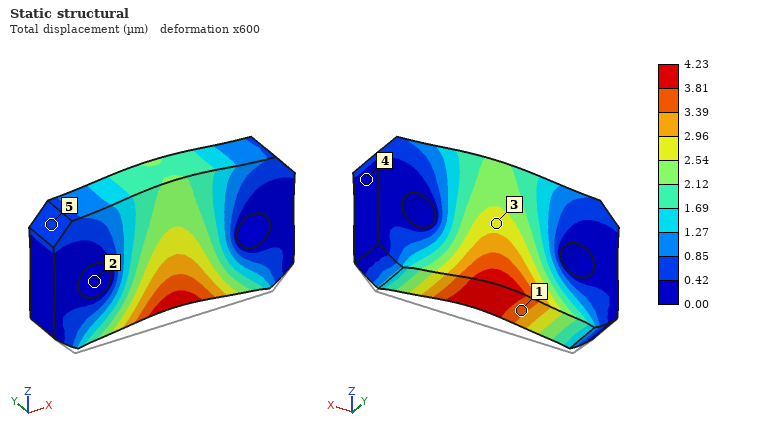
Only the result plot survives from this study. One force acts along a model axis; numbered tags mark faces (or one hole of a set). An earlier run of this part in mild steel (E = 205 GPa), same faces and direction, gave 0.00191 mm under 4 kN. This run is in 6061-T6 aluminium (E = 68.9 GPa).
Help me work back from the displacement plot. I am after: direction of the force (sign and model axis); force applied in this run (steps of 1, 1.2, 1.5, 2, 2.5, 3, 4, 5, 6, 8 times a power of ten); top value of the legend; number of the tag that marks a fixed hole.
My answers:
+Z
3 kN
4.23 µm
2
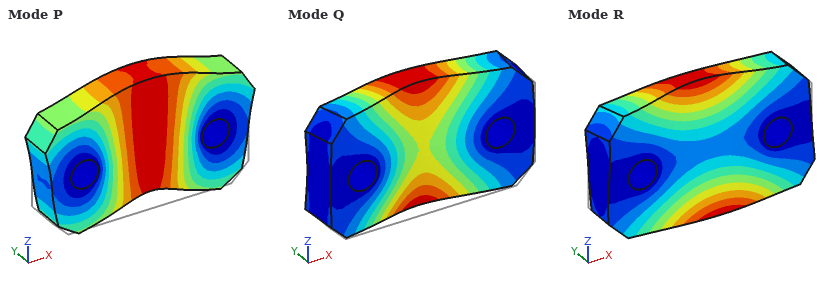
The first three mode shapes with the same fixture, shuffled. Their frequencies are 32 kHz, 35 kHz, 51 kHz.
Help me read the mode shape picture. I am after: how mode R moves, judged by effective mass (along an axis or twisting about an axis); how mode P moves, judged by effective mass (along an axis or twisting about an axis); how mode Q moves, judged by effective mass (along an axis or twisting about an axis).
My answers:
twisting about X
along Z
along Y
